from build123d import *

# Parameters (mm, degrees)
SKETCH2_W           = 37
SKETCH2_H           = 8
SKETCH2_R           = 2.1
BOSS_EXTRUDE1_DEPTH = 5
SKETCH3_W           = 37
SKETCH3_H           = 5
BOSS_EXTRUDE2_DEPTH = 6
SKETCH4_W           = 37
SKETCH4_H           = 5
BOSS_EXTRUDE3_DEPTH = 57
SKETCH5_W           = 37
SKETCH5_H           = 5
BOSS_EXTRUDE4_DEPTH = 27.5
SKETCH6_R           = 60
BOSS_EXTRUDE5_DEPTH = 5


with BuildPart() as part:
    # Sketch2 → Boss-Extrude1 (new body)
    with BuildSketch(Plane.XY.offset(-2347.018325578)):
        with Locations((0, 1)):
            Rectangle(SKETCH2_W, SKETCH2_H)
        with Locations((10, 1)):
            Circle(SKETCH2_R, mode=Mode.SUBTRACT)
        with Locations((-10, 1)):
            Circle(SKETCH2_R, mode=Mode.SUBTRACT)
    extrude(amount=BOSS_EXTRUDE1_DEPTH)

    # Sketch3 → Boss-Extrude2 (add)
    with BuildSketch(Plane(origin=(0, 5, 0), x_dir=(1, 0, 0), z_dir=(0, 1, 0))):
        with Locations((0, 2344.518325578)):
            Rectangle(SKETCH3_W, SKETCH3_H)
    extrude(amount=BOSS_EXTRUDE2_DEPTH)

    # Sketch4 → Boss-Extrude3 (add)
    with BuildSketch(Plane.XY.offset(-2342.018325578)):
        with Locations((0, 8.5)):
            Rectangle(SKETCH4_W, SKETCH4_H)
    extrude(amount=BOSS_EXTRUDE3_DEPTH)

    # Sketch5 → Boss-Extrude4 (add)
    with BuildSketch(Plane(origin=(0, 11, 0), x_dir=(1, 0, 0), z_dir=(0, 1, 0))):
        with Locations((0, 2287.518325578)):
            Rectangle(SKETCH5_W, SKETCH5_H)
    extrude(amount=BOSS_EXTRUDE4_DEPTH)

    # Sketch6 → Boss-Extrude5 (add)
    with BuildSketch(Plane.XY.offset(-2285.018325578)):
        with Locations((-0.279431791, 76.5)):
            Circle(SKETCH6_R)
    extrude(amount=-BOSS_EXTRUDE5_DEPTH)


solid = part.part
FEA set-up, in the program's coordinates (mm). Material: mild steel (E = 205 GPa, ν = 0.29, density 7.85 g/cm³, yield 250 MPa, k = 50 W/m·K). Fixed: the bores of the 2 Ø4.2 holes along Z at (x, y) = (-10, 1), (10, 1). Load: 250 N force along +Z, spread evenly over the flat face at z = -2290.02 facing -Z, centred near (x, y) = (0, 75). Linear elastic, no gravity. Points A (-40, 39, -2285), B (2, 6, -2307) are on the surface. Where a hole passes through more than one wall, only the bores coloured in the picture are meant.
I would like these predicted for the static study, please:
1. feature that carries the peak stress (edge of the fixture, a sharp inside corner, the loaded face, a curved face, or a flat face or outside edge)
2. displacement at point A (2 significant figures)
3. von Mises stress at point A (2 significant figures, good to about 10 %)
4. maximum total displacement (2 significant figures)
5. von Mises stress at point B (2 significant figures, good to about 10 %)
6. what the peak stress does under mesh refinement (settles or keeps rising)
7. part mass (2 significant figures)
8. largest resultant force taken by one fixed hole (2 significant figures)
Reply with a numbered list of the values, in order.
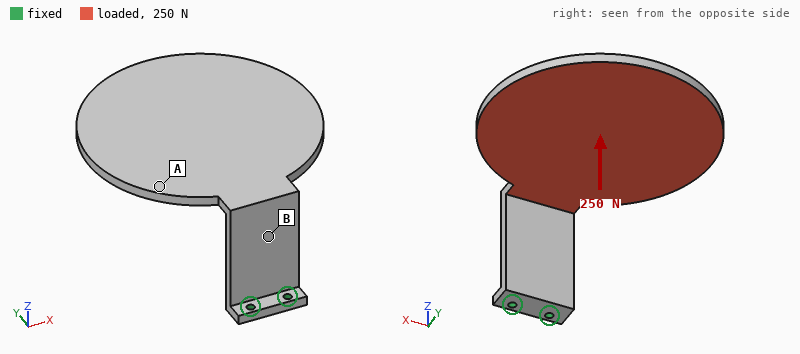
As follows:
1. edge of the fixture
2. 0.66 mm
3. 16 MPa
4. 2.2 mm
5. 98 MPa
6. keeps rising
7. 560 g
8. 210 N
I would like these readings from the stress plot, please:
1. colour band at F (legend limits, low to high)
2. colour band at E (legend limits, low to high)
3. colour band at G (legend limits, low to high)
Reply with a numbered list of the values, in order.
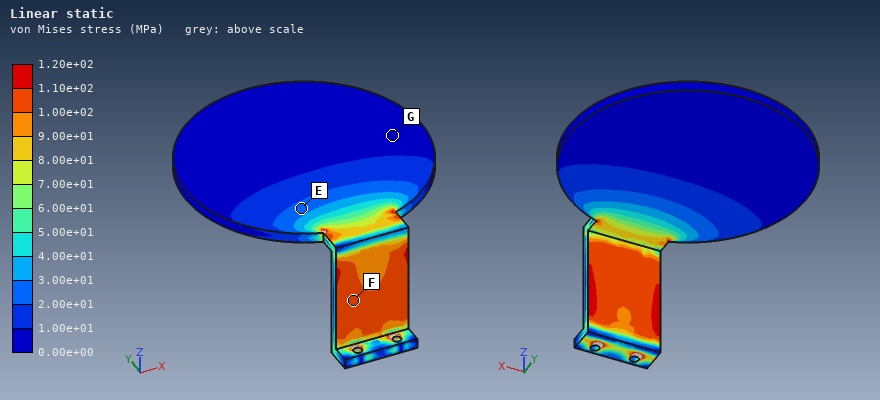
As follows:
1. 1.00e+02 to 1.10e+02 MPa
2. 2.00e+01 to 3.00e+01 MPa
3. 0.00e+00 to 1.00e+01 MPa
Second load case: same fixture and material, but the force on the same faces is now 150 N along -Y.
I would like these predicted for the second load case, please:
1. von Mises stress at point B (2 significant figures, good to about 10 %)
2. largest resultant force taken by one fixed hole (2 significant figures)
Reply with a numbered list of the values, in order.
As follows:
1. 16 MPa
2. 100 N
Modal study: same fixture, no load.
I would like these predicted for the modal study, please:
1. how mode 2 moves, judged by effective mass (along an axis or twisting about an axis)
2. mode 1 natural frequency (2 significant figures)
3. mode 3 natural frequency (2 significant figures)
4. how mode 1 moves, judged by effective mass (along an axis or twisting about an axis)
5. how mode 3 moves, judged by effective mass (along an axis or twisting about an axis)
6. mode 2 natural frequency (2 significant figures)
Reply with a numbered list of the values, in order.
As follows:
1. along X
2. 95 Hz
3. 370 Hz
4. along Z
5. along Y
6. 150 Hz
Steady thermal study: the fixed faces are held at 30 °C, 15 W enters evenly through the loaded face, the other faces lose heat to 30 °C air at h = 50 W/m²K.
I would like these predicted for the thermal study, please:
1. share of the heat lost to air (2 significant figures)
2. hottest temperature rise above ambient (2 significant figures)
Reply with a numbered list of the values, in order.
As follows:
1. 92 %
2. 20 K
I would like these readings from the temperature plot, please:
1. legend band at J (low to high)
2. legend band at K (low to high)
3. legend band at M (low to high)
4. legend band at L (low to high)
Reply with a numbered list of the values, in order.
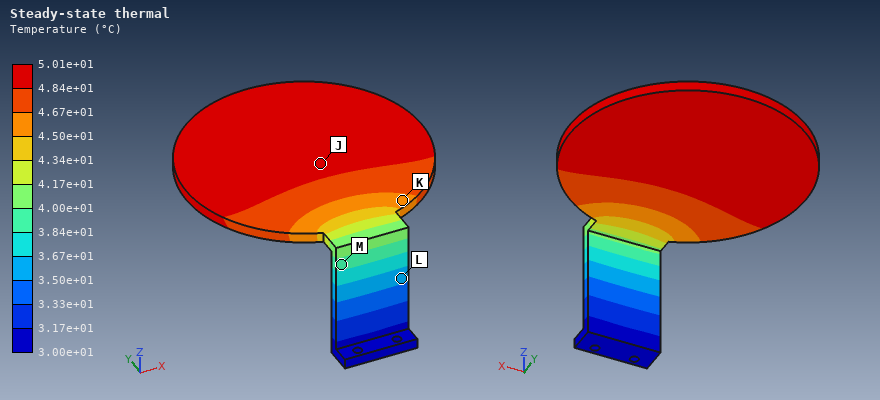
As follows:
1. 4.84e+01 to 5.01e+01 °C
2. 4.50e+01 to 4.67e+01 °C
3. 3.84e+01 to 4.00e+01 °C
4. 3.50e+01 to 3.67e+01 °C
